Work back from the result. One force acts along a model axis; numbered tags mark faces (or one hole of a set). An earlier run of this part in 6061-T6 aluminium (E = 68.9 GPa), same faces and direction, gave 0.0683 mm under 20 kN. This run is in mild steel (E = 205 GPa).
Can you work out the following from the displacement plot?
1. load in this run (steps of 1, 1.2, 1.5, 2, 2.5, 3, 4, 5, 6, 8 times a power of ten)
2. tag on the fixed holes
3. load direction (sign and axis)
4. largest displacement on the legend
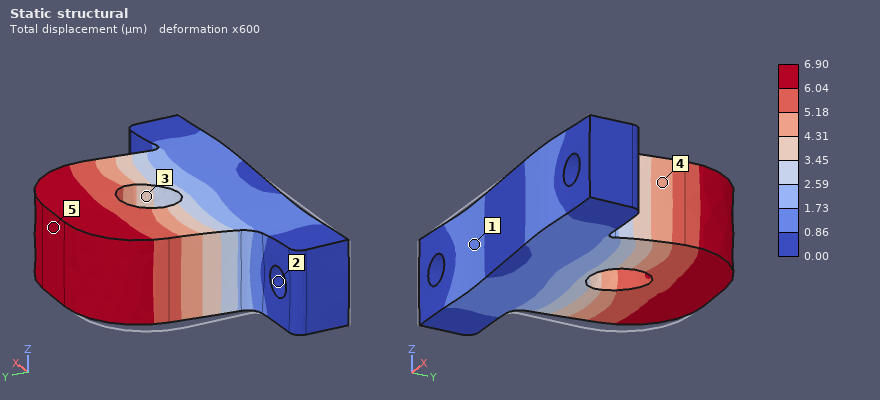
6 kN
2
+X
6.90 µm
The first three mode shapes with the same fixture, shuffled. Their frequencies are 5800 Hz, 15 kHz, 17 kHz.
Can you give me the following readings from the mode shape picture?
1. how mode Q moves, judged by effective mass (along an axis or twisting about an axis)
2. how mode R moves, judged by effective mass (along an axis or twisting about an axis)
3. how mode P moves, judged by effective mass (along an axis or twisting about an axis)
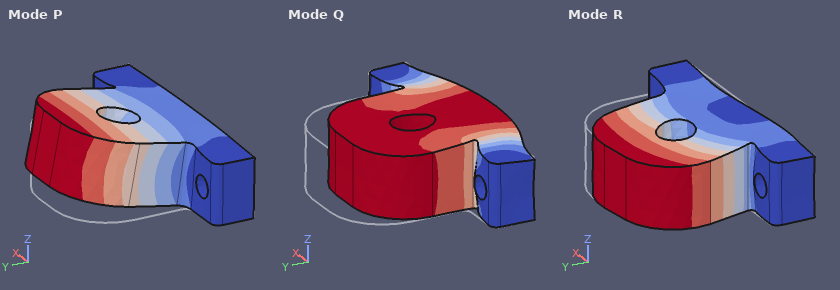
along Y
along X
along Z
